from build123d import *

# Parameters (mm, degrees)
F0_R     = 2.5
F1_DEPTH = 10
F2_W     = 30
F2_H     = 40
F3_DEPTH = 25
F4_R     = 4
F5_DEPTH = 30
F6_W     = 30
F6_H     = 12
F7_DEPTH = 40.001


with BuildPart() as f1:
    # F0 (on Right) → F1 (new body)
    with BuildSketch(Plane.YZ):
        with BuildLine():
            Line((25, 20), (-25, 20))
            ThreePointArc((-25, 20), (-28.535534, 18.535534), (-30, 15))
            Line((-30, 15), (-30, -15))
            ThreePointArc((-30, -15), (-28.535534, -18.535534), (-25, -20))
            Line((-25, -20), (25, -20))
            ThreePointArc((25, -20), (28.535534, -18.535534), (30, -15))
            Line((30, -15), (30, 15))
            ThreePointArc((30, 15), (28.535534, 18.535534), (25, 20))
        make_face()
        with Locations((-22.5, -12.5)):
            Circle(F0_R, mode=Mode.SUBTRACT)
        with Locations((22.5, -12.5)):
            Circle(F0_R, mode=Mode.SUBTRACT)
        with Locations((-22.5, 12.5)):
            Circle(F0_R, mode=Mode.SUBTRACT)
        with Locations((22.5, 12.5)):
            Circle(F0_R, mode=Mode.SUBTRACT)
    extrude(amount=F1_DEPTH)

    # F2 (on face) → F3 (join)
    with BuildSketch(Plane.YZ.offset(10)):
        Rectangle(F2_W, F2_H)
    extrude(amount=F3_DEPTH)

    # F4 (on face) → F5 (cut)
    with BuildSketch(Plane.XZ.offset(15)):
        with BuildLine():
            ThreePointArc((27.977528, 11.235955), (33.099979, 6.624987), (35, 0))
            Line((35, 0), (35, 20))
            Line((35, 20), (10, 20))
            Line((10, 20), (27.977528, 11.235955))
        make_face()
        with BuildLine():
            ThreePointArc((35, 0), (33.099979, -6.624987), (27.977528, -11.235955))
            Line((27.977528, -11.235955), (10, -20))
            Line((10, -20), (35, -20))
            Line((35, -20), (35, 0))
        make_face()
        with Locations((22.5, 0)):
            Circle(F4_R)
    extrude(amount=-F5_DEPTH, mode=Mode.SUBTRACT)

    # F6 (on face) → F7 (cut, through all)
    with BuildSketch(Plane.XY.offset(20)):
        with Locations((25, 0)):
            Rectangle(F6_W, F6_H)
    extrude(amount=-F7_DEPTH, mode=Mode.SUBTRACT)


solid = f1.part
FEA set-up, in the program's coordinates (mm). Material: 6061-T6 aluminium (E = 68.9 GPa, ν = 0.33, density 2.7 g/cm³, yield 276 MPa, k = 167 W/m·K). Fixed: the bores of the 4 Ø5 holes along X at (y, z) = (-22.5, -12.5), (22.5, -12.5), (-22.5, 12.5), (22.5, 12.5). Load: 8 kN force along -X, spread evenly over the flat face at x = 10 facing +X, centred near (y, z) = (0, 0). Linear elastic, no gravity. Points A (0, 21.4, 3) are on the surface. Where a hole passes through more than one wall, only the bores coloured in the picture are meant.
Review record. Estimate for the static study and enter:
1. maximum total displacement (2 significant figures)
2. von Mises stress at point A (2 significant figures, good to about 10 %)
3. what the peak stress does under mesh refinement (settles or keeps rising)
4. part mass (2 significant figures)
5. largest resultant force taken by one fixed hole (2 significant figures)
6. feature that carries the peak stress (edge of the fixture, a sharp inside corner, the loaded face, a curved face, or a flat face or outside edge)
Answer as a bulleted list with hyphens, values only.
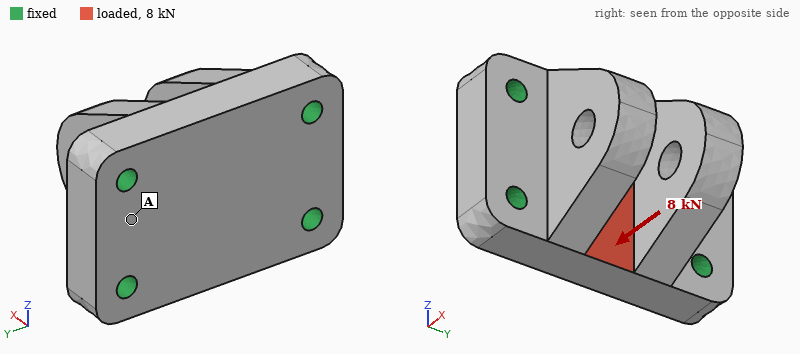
- 43 µm
- 16 MPa
- keeps rising
- 92 g
- 2.0 kN
- edge of the fixture
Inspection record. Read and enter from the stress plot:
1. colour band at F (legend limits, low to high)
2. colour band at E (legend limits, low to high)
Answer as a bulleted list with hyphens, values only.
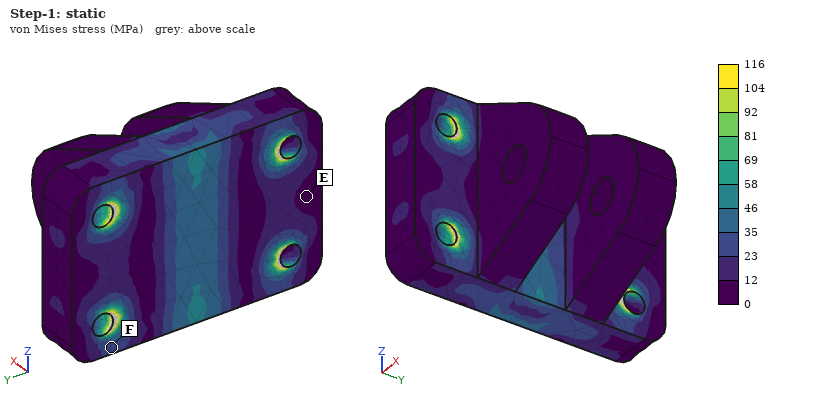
- 23 to 35 MPa
- 0 to 12 MPa
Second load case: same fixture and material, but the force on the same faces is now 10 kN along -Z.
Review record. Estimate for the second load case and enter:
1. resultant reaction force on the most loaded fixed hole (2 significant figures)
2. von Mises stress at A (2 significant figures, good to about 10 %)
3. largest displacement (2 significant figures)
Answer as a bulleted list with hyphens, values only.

- 3.1 kN
- 8.5 MPa
- 21 µm
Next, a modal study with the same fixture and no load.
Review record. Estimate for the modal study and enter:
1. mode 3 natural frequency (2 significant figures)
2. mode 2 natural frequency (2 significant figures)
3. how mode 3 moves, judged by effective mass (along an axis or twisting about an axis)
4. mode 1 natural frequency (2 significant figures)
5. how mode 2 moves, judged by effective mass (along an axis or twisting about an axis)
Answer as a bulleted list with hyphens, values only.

- 14 kHz
- 12 kHz
- along Z
- 9600 Hz
- along Y
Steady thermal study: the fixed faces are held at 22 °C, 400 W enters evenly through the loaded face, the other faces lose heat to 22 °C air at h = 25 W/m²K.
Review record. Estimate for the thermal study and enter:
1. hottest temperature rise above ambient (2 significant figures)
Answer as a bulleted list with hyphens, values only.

- 70 K
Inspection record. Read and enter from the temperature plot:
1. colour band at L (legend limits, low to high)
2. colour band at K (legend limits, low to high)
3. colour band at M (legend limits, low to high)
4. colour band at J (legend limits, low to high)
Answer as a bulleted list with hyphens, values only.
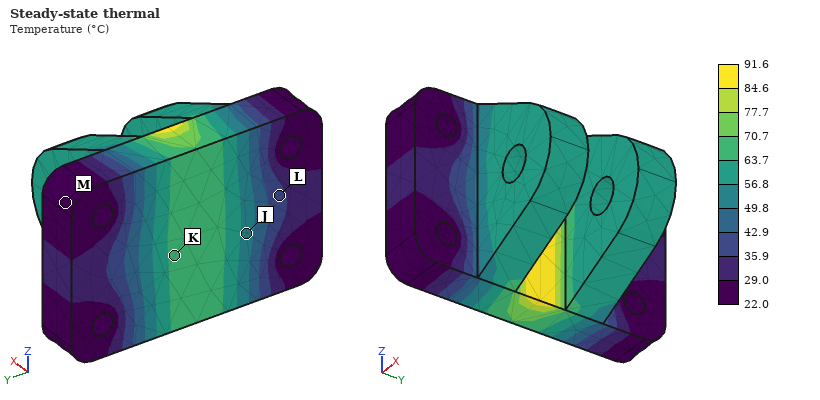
- 35.9 to 42.9 °C
- 63.7 to 70.7 °C
- 22.0 to 29.0 °C
- 49.8 to 56.8 °C
